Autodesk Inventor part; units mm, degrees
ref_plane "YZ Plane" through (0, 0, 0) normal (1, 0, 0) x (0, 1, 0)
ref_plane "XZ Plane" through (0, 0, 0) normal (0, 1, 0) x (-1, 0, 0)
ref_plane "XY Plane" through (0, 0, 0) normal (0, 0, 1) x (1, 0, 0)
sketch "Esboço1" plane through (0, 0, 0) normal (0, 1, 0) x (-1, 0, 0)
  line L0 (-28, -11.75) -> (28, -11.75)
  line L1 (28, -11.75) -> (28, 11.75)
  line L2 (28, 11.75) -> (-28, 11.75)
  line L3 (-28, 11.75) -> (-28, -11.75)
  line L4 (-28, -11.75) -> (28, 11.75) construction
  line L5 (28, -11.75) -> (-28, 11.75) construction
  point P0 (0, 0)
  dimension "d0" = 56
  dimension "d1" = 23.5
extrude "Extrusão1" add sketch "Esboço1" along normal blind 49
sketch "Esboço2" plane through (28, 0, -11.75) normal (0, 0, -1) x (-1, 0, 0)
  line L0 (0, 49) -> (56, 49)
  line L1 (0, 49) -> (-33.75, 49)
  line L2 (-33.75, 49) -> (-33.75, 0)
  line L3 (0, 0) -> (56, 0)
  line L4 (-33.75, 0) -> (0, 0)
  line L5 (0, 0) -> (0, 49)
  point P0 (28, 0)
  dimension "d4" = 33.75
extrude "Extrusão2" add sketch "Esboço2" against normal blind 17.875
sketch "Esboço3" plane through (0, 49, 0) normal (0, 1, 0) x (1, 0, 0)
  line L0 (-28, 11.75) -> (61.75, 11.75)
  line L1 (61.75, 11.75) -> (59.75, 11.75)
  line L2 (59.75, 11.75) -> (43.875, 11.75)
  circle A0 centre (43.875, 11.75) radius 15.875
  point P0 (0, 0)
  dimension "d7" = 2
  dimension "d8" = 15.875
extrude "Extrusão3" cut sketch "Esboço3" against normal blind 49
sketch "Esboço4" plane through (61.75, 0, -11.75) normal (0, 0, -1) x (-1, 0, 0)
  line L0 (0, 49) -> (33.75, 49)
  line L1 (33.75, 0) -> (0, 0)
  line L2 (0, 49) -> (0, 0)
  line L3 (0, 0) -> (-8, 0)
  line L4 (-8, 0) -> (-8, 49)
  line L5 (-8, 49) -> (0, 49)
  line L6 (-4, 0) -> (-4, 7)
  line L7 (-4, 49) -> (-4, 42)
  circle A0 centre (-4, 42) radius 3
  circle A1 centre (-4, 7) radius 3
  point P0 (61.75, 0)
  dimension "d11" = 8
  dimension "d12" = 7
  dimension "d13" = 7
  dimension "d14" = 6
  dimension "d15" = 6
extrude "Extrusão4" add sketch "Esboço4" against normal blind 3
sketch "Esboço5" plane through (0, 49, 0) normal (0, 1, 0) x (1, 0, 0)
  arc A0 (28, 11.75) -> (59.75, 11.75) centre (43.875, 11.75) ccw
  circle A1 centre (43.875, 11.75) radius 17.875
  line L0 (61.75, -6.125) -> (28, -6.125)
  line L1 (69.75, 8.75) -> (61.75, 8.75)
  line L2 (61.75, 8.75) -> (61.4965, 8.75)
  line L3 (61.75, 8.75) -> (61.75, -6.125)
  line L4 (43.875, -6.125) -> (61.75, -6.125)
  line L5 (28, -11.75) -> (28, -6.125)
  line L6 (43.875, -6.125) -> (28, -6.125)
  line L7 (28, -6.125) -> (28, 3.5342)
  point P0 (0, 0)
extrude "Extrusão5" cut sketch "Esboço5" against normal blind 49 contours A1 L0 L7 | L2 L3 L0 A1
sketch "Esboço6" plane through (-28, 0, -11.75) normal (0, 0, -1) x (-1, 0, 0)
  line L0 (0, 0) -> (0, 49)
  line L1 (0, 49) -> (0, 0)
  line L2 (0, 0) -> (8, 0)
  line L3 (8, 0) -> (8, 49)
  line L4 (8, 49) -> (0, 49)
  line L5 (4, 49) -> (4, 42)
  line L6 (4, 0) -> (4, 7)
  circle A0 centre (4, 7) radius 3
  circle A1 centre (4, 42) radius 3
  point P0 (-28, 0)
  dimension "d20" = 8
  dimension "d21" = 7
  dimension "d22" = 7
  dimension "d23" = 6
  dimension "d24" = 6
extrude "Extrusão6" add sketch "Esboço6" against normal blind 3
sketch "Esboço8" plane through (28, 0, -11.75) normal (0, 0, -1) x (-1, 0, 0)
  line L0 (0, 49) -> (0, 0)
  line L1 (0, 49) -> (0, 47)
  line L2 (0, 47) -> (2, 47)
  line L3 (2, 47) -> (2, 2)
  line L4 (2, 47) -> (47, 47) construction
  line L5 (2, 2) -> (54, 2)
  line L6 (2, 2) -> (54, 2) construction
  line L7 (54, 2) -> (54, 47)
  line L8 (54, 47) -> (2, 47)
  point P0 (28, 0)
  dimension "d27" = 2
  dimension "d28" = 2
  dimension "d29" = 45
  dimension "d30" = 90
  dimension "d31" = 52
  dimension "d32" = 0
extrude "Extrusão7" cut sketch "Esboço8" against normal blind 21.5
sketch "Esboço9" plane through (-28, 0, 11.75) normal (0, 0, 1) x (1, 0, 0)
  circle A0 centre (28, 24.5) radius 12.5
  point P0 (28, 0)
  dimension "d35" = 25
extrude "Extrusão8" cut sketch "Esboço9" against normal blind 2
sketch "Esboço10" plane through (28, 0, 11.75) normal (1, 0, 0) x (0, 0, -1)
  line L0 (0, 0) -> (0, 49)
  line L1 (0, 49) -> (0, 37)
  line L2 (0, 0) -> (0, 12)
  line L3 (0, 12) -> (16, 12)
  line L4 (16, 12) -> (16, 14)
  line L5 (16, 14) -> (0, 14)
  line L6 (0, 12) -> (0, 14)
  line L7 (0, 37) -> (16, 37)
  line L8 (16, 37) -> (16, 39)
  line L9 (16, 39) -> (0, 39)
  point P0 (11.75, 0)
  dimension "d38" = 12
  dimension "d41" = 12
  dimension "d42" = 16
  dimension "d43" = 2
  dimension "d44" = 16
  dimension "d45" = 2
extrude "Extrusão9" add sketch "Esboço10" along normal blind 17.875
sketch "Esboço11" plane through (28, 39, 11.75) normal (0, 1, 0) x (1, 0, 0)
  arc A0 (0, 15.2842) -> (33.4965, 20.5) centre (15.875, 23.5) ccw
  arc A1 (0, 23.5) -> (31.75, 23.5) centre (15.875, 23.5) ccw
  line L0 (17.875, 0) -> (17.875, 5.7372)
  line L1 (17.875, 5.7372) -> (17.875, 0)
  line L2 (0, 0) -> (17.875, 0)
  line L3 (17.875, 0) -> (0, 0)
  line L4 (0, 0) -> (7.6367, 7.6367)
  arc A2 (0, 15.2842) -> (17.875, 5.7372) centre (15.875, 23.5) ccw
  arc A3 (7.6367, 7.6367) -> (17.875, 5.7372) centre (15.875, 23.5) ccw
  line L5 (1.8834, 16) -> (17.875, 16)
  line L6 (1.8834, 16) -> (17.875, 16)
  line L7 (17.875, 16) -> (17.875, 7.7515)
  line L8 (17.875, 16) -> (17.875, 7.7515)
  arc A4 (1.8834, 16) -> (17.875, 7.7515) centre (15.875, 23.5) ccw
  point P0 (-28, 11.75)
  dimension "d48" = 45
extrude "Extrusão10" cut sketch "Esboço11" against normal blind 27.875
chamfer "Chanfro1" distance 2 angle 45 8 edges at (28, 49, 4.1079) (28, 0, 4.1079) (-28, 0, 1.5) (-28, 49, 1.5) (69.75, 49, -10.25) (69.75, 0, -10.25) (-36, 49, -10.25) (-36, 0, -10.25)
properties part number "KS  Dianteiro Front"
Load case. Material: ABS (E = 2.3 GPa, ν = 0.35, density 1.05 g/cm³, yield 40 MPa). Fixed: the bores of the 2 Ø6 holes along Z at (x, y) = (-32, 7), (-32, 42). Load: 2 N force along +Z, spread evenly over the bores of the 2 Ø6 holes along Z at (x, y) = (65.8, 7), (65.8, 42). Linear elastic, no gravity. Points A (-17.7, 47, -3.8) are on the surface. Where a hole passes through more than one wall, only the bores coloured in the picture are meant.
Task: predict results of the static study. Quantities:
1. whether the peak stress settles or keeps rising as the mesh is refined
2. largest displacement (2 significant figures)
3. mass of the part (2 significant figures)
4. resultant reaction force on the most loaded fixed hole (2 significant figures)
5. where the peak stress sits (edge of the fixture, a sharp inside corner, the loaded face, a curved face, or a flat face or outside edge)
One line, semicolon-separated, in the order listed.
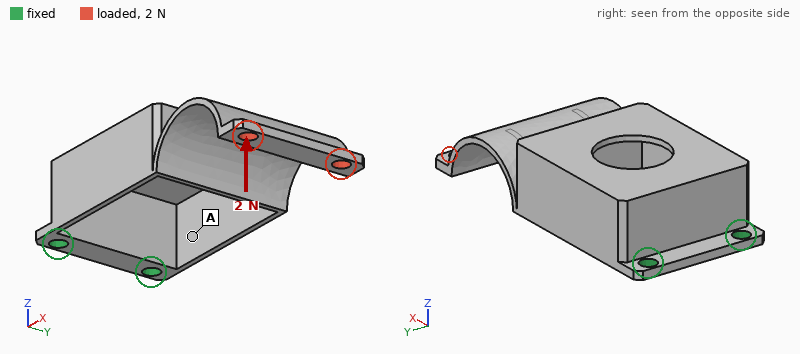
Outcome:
keeps rising; 1.3 mm; 21 g; 2.4 N; a sharp inside corner
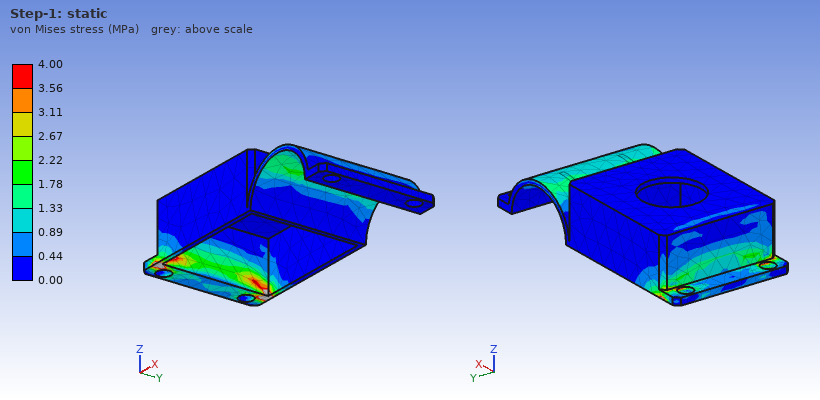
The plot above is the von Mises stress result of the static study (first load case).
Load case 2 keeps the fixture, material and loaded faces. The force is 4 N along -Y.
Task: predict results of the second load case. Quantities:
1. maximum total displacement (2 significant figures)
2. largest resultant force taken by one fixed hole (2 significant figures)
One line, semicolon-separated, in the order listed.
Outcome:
1.2 mm; 8.5 N
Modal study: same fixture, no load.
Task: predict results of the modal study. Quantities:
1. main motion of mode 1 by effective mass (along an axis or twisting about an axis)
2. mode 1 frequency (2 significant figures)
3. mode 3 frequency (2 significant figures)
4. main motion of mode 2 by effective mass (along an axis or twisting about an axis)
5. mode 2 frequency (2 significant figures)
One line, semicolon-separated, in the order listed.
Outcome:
along Z; 92 Hz; 310 Hz; along Y; 130 Hz
